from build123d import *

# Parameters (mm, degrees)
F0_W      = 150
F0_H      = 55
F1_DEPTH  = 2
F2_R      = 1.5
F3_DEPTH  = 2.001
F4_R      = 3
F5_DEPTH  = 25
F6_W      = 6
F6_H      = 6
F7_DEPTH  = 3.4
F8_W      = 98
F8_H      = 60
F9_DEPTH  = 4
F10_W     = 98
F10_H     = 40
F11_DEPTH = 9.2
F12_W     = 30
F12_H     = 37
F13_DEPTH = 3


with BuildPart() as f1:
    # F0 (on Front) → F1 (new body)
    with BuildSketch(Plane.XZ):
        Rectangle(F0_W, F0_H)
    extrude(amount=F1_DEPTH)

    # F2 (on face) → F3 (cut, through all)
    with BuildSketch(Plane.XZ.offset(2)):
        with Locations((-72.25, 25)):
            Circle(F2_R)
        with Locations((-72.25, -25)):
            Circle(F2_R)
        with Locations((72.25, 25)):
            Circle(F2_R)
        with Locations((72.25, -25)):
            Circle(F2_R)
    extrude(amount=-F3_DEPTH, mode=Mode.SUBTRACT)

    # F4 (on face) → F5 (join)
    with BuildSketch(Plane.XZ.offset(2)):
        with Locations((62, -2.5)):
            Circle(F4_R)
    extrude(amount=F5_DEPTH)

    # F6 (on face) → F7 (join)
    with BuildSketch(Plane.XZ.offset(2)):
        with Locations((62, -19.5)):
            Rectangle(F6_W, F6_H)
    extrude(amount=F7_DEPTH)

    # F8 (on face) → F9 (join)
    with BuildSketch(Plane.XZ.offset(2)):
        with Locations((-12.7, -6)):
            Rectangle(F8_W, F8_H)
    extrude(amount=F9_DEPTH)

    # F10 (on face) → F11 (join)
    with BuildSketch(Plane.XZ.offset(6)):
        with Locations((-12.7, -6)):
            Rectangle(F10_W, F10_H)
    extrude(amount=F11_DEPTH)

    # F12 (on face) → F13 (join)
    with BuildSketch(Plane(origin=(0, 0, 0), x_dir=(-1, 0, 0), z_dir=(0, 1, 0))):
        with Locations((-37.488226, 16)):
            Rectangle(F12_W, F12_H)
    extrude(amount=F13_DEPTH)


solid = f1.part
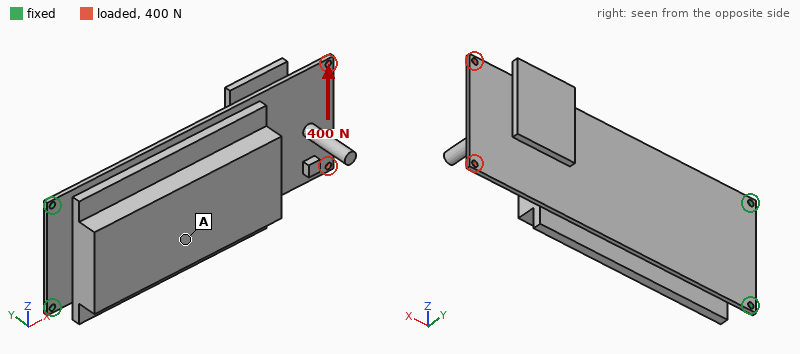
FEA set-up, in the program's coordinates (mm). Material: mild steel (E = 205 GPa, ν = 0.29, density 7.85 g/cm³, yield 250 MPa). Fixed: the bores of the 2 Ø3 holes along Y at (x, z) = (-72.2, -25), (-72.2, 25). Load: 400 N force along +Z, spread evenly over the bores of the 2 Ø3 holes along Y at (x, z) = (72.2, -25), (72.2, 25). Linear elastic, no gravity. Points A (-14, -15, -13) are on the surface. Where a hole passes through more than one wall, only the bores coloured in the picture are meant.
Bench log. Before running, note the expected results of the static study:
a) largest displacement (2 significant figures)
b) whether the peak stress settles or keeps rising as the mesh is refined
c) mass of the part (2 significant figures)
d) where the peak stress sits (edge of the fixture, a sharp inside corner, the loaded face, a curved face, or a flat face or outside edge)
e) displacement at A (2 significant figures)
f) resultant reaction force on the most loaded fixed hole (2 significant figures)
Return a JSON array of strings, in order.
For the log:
["51 µm", "keeps rising", "630 g", "edge of the fixture", "11 µm", "1.2 kN"]
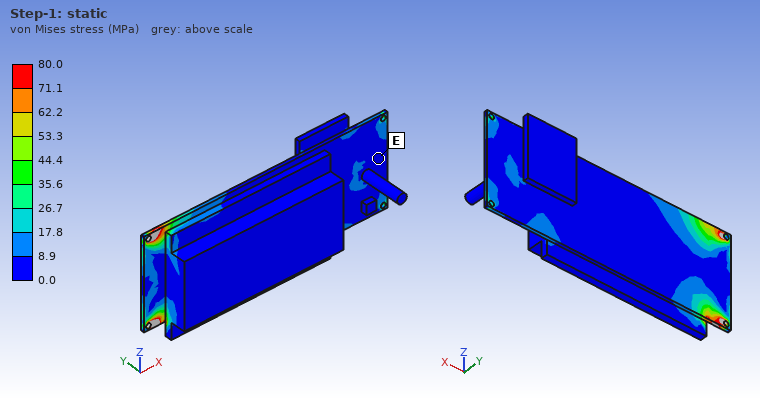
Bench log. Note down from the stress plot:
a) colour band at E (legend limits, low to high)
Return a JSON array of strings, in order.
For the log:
["0.0 to 8.9 MPa"]
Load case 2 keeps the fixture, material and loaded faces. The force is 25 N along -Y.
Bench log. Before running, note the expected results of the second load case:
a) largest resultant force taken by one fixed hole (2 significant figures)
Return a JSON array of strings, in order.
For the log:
["14 N"]
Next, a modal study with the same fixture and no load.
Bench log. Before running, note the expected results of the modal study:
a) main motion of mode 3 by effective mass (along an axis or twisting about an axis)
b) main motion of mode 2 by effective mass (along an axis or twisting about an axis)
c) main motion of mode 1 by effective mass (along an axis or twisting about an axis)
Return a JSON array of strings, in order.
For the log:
["along Z", "along Z", "along Y"]
